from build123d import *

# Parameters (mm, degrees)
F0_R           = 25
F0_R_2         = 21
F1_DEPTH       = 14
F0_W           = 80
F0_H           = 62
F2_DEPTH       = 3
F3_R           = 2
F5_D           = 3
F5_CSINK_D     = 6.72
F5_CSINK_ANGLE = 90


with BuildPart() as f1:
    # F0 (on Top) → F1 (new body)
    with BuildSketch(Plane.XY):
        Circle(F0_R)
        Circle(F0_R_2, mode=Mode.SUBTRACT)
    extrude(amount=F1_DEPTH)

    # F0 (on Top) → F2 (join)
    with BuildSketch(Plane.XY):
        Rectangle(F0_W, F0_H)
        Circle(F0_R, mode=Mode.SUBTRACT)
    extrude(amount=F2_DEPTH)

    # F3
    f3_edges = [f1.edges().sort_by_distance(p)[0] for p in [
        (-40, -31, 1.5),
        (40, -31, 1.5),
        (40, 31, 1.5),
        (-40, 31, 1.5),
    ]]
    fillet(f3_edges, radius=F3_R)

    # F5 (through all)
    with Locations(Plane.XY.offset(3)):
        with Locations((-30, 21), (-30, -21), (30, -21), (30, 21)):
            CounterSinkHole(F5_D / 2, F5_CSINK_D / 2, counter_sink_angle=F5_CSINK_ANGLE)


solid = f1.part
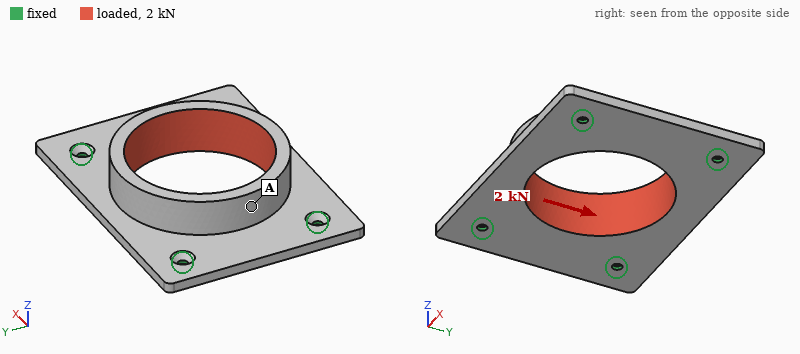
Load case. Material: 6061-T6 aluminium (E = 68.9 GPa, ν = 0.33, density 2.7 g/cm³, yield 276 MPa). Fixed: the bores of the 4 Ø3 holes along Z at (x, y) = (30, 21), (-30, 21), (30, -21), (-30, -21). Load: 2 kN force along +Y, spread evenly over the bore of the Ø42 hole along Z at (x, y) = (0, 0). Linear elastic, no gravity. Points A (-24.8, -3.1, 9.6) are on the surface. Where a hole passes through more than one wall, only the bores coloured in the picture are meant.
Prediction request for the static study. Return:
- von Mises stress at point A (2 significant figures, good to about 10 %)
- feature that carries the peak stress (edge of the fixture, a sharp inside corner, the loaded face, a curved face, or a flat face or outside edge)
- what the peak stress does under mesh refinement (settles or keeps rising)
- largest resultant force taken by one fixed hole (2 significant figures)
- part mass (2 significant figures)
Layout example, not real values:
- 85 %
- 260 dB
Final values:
- 8.3 MPa
- edge of the fixture
- keeps rising
- 560 N
- 46 g
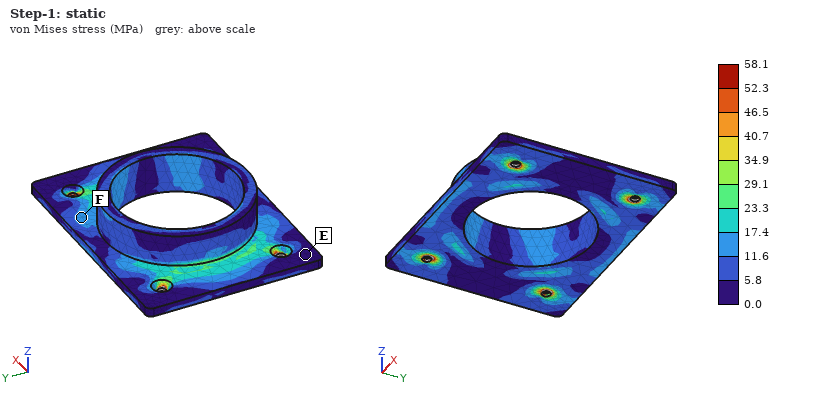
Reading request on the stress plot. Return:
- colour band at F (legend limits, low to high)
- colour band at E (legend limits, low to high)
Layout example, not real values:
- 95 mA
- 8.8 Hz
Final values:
- 11.6 to 17.4 MPa
- 0.0 to 5.8 MPa
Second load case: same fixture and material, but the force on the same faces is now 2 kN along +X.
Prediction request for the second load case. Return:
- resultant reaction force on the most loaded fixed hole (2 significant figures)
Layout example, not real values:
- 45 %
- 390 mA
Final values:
- 520 N
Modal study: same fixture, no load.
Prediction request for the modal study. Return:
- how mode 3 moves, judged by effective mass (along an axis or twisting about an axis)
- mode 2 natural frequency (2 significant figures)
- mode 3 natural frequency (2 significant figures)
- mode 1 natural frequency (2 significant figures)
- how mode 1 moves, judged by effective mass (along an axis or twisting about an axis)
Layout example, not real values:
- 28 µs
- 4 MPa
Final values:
- twisting about Y
- 4800 Hz
- 7000 Hz
- 4300 Hz
- along Z
